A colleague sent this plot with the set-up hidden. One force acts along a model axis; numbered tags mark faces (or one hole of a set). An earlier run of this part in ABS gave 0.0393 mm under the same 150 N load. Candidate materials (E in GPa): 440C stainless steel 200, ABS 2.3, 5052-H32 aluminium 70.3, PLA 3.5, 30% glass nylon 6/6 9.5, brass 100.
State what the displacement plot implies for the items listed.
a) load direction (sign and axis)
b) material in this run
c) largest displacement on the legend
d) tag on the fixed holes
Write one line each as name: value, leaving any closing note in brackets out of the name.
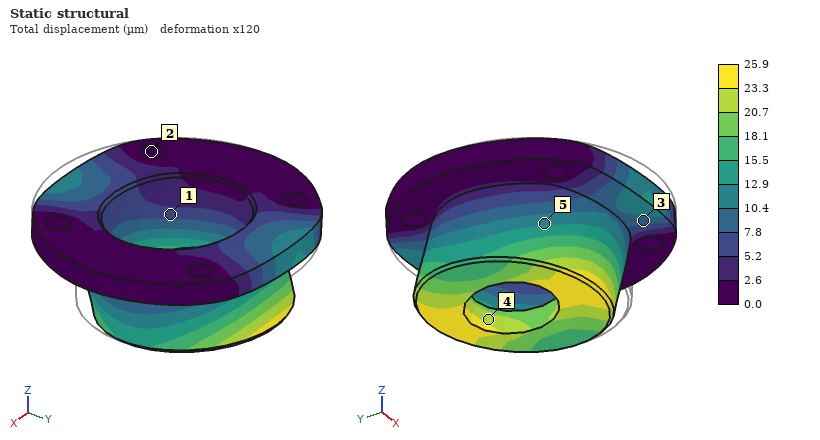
load direction: +Y
material in this run: PLA
largest displacement on the legend: 25.9 µm
tag on the fixed holes: 2
